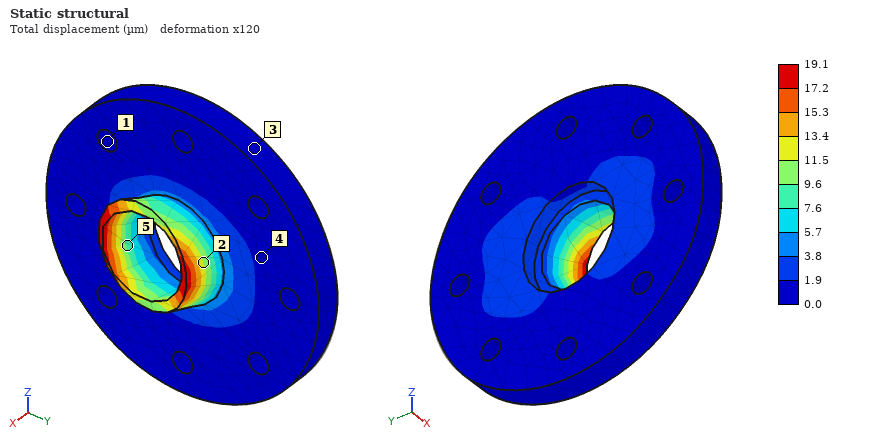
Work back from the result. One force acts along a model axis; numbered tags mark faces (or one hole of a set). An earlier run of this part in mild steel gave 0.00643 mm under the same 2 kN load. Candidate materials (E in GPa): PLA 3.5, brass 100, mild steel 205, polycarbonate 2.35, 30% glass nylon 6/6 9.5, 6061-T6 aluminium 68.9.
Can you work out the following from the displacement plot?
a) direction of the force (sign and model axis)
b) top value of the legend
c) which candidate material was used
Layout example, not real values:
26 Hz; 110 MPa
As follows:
-Y; 19.1 µm; 6061-T6 aluminium
